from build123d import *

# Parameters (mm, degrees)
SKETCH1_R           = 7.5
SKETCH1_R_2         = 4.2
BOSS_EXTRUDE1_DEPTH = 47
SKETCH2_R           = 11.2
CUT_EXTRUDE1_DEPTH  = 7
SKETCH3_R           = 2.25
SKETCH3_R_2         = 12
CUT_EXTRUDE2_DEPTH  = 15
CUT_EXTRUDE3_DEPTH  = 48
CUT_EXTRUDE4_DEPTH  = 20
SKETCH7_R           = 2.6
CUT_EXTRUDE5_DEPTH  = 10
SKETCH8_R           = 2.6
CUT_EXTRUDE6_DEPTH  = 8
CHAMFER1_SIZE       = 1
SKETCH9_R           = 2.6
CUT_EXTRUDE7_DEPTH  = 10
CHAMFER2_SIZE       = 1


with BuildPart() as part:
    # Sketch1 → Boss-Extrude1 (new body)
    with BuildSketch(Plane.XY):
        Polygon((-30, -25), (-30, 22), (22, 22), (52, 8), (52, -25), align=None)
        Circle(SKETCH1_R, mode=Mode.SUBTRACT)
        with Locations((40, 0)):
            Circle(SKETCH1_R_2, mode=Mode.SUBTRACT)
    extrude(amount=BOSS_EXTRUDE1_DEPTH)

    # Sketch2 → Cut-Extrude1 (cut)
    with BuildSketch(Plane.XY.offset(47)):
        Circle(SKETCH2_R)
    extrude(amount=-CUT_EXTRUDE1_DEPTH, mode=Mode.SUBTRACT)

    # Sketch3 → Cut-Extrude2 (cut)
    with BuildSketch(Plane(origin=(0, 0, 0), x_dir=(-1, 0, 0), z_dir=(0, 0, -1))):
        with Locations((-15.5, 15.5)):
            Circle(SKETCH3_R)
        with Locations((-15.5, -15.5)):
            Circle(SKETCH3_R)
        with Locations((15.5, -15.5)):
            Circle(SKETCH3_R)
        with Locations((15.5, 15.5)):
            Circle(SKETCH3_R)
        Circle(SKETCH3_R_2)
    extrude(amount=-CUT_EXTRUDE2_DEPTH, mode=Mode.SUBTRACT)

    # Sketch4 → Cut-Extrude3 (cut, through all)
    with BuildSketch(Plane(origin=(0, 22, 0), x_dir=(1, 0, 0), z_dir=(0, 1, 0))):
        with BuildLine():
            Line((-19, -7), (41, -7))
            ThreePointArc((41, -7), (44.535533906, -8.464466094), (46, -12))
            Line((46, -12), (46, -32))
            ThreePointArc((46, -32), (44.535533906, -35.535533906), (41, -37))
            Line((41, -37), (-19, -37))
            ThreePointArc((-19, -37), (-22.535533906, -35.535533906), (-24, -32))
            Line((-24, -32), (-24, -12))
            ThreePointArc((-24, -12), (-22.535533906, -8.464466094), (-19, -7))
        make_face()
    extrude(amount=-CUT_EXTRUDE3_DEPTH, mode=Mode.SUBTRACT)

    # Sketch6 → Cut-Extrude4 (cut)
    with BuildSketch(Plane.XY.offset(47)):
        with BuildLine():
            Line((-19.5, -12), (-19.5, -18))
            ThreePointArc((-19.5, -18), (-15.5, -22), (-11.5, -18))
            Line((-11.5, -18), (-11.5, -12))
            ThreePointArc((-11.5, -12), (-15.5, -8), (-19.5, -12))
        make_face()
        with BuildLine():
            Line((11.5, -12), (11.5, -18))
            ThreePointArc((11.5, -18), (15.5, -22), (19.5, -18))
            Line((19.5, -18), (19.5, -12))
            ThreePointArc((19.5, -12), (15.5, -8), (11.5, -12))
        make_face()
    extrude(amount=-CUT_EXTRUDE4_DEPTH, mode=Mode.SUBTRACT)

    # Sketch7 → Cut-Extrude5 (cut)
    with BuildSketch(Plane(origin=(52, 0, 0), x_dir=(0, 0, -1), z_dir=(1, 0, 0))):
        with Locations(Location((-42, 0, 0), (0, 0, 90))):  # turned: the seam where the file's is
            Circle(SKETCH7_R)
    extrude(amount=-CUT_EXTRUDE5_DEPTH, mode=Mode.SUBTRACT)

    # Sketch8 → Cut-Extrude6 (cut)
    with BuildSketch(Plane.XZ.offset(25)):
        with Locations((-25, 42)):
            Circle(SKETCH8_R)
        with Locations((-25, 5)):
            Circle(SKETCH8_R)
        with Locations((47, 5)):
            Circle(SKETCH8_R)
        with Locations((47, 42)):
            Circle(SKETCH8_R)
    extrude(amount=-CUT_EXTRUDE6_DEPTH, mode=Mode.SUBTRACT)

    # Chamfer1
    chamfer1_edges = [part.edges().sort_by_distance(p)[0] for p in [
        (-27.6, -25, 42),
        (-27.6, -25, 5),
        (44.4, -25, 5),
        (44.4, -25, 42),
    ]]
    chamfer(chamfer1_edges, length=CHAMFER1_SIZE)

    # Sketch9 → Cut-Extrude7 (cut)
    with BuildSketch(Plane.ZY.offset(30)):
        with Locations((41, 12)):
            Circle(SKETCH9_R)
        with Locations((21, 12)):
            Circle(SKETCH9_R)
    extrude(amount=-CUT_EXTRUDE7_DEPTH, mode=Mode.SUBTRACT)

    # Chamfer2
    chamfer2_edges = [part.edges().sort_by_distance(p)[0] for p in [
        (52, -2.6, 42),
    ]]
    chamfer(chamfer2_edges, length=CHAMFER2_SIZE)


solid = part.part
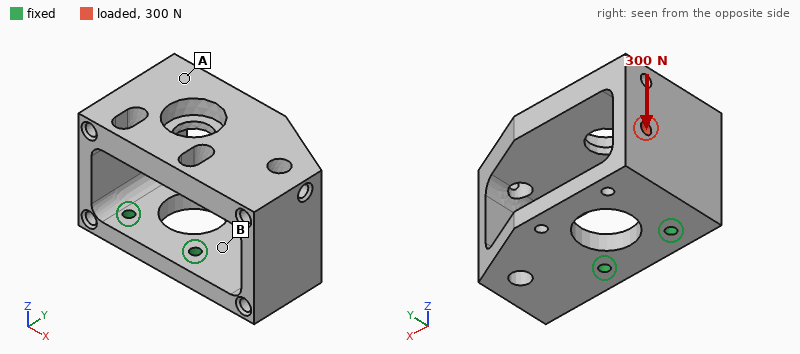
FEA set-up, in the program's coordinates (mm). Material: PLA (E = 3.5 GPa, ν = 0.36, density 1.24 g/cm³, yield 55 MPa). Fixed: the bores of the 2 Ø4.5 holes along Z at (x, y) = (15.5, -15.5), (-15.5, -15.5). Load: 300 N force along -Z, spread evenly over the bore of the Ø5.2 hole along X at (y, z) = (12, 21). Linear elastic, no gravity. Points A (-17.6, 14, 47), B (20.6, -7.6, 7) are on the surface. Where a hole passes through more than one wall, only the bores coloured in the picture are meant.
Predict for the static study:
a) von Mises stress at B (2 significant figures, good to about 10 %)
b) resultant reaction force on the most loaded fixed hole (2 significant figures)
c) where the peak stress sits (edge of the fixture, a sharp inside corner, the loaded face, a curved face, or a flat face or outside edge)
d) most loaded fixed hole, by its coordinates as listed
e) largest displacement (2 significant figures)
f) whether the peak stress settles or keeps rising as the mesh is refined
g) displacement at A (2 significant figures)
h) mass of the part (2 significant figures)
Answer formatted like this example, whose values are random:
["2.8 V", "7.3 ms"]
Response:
["6.9 MPa", "320 N", "edge of the fixture", "(-15.5, -15.5)", "1.1 mm", "keeps rising", "0.98 mm", "82 g"]
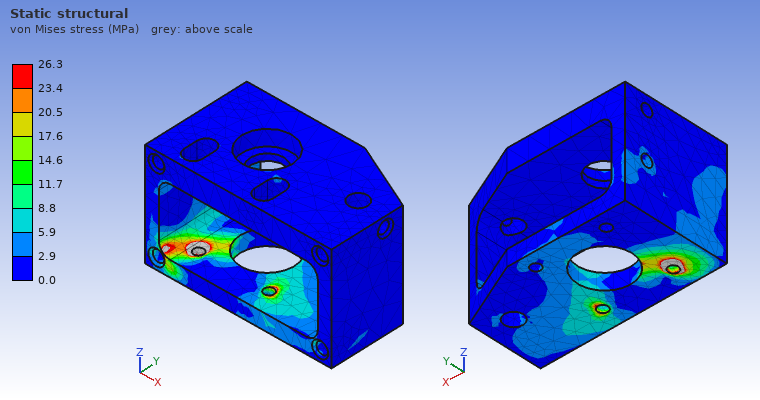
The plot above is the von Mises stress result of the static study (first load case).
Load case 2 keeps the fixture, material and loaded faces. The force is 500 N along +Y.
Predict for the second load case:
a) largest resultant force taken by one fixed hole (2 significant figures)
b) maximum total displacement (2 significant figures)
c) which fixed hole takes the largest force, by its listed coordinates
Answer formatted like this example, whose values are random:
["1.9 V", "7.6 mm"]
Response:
["610 N", "1.2 mm", "(-15.5, -15.5)"]
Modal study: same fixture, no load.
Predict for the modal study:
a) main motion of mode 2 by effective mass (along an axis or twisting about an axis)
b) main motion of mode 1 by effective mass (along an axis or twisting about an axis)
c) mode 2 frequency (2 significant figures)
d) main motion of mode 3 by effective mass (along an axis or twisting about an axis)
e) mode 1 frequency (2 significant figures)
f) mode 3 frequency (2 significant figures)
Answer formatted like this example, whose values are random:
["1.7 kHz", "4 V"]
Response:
["along X", "along Y", "400 Hz", "along Z", "350 Hz", "830 Hz"]
